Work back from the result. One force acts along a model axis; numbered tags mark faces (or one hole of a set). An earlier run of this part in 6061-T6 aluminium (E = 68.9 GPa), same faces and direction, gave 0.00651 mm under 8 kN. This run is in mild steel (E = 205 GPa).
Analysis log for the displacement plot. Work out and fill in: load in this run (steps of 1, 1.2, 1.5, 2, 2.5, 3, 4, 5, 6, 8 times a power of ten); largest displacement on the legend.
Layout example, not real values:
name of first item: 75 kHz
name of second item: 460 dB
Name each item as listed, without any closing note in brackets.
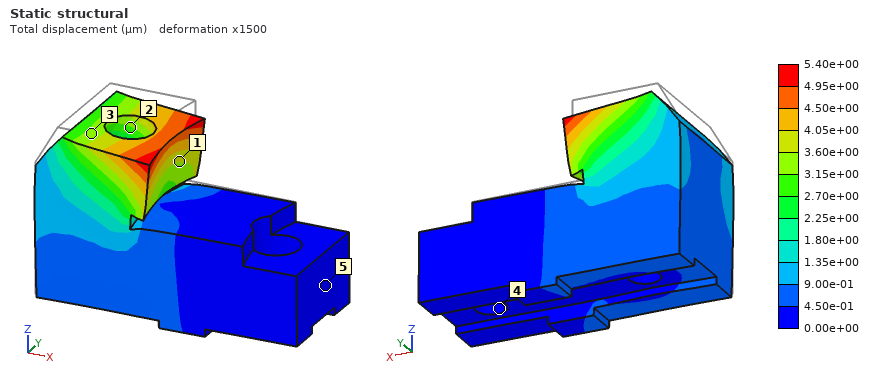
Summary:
load in this run: 20 kN
largest displacement on the legend: 5.40e+00 µm
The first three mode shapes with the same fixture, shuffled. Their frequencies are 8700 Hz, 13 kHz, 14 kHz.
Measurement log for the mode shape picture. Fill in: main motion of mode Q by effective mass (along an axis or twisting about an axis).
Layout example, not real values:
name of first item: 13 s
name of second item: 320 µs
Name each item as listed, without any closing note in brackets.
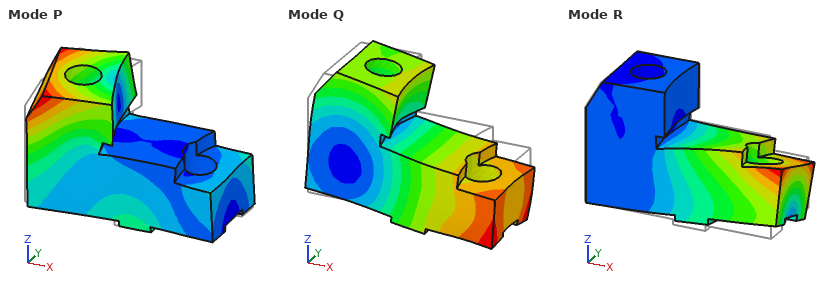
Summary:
main motion of mode Q by effective mass: along Z
